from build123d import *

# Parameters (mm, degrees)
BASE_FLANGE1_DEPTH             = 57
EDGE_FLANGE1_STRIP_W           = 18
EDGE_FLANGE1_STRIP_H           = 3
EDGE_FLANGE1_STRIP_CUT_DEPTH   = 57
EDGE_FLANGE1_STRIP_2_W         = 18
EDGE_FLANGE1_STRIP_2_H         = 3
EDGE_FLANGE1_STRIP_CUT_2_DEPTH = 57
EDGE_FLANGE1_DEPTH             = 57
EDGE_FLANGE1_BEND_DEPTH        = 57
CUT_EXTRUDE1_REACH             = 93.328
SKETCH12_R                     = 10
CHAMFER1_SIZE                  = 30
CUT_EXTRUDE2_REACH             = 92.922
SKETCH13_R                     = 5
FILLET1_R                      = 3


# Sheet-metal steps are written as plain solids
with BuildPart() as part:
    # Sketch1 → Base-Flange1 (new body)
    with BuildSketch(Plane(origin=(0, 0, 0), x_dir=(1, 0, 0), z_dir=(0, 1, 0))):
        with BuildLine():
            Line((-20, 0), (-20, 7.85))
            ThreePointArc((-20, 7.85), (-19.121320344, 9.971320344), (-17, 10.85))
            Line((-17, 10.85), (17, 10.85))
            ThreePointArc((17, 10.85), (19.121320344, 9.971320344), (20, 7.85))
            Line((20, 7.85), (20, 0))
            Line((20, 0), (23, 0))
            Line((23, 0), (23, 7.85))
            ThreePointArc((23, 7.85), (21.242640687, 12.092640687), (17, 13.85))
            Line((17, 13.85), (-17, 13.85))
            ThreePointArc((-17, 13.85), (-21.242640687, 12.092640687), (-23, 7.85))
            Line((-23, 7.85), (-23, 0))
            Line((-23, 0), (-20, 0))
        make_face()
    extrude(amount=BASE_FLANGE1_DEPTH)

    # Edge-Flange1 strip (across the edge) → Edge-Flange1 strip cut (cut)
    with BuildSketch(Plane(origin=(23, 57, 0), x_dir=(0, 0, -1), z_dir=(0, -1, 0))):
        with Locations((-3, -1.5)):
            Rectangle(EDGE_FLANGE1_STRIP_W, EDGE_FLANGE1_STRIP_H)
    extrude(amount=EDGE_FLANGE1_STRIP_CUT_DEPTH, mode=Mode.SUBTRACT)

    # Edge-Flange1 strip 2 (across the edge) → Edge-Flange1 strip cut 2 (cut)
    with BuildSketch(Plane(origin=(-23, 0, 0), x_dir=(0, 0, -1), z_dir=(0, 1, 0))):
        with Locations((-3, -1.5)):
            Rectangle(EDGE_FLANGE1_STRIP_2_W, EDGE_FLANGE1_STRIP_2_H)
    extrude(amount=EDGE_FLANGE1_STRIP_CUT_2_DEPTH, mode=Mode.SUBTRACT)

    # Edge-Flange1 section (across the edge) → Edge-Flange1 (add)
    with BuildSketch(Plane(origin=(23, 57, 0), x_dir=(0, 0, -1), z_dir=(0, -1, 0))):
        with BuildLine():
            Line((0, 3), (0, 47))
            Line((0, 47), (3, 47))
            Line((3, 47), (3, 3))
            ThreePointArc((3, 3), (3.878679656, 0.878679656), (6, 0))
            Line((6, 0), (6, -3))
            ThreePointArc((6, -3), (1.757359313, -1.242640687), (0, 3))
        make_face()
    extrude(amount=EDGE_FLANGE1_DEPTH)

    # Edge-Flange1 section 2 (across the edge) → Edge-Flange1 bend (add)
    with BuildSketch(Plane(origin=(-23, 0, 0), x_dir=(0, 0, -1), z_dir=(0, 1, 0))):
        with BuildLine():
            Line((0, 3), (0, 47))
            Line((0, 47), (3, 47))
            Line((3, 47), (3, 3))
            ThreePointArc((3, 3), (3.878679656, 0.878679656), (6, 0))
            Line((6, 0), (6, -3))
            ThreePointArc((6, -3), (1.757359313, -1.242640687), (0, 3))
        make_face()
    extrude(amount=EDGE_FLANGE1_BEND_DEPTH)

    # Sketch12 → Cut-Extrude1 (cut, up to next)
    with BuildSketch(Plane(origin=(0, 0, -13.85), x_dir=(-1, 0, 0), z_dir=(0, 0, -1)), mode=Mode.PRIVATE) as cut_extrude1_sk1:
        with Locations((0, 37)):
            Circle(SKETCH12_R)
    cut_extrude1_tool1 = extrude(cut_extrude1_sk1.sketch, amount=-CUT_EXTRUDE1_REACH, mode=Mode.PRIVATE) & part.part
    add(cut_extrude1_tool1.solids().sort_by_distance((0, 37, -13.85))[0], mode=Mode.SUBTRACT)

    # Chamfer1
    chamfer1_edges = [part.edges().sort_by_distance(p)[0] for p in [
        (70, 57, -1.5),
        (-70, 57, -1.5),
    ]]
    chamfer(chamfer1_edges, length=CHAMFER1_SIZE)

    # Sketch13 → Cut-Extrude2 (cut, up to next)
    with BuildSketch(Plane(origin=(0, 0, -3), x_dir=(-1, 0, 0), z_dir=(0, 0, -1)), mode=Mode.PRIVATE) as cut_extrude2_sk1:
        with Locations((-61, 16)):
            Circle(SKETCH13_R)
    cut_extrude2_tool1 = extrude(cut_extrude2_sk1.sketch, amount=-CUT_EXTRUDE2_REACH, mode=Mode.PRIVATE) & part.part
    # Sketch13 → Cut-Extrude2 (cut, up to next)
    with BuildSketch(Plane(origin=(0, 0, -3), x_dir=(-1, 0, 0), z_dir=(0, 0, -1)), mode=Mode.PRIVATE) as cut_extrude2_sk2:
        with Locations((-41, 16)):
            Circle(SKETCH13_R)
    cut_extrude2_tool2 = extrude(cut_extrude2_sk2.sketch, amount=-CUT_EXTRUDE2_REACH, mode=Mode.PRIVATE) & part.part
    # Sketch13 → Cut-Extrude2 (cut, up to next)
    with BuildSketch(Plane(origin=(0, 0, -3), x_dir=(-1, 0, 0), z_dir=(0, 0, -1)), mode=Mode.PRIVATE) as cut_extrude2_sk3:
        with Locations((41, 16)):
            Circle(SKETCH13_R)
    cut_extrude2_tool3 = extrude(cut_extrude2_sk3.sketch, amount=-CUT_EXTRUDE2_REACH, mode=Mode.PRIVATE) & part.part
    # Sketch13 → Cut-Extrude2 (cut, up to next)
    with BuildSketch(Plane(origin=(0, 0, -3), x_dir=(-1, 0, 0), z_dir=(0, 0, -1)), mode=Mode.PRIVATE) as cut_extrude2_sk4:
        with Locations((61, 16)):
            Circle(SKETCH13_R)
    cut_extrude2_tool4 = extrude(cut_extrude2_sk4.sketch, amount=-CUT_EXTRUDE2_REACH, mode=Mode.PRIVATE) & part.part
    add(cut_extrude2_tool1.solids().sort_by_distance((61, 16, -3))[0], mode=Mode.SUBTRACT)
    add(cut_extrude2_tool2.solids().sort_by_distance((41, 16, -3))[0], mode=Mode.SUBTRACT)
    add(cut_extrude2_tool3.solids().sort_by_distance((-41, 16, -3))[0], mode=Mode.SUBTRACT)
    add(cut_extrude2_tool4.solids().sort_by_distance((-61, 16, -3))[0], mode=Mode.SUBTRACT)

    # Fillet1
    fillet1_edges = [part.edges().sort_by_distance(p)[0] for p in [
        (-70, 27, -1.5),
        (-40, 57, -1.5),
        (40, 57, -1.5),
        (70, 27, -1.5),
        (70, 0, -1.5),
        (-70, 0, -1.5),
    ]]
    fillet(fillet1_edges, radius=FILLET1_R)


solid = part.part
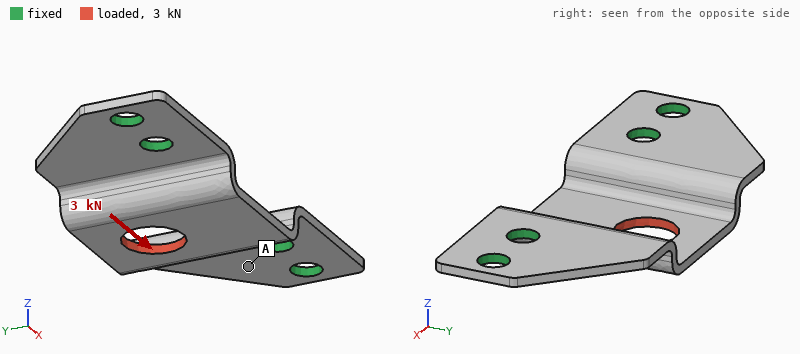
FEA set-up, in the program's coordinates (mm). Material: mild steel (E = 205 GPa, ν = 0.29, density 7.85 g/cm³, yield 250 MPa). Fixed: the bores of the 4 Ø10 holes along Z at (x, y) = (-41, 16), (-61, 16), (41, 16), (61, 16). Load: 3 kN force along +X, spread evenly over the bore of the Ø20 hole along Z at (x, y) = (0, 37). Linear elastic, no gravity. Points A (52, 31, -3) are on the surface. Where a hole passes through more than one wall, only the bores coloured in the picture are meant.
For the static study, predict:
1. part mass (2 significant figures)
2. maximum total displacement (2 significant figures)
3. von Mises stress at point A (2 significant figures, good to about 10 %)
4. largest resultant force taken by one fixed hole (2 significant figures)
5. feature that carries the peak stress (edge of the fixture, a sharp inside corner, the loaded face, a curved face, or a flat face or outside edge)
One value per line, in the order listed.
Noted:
170 g
43 µm
13 MPa
1.2 kN
a curved face
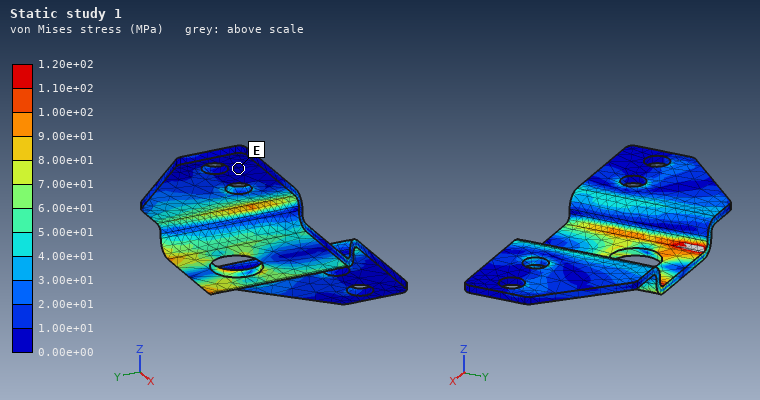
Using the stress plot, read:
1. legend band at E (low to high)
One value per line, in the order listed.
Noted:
0.00e+00 to 1.00e+01 MPa
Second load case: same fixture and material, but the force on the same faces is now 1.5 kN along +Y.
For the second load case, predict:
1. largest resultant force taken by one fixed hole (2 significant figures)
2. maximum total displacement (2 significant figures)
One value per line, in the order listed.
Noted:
1.3 kN
0.11 mm
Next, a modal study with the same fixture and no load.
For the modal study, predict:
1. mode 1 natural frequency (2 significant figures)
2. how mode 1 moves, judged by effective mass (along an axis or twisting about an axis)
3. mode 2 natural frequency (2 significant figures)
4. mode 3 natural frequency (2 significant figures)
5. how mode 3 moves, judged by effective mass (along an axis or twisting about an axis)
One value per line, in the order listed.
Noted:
1700 Hz
along Z
3500 Hz
4900 Hz
along Z
